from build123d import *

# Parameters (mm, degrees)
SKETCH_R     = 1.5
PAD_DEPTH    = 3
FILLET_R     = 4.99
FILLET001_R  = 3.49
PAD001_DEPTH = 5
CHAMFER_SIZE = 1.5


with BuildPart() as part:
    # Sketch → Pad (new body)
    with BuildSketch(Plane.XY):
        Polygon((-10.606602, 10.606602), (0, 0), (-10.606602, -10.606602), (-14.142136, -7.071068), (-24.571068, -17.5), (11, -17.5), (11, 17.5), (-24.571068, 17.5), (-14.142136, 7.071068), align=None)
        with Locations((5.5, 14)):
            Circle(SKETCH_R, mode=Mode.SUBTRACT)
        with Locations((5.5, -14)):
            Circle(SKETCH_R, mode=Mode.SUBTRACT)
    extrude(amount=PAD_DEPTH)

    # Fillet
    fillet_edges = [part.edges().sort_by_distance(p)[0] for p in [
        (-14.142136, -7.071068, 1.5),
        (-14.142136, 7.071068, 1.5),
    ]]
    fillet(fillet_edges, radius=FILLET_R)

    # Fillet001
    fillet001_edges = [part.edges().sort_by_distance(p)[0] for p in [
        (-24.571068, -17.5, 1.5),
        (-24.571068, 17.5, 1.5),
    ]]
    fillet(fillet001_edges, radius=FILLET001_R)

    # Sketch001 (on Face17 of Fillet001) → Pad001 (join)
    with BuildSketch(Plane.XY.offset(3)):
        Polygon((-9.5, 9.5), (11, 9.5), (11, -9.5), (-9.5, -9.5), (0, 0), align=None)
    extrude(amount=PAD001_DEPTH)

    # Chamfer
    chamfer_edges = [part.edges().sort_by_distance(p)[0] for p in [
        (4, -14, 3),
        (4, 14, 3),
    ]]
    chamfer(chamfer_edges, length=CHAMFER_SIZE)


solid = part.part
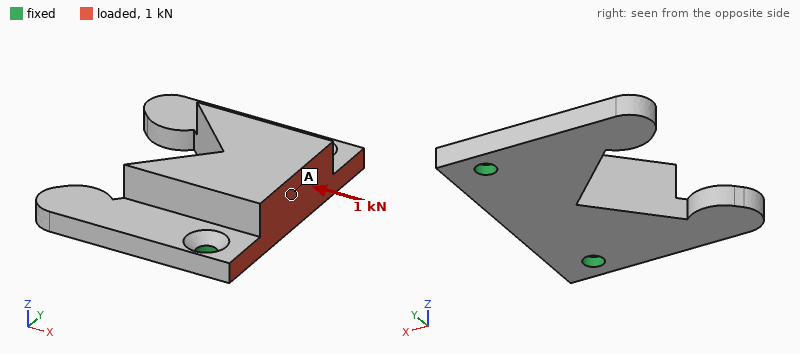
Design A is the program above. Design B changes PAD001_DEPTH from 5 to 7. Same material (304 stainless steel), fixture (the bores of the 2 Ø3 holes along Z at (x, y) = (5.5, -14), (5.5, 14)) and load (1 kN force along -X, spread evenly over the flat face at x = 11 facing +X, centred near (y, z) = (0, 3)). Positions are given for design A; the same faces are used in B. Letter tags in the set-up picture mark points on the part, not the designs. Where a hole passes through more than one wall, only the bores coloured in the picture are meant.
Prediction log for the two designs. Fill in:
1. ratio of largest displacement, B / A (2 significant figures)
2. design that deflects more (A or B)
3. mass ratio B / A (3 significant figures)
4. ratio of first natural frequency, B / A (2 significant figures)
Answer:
1.4
B
1.16
0.94
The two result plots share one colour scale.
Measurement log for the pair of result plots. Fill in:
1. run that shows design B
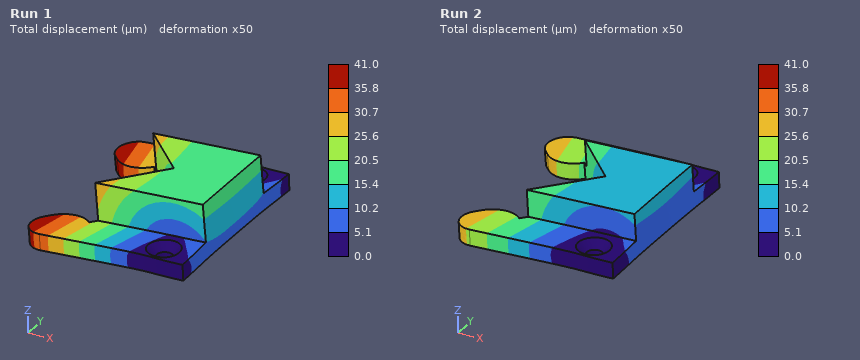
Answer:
Run 1
